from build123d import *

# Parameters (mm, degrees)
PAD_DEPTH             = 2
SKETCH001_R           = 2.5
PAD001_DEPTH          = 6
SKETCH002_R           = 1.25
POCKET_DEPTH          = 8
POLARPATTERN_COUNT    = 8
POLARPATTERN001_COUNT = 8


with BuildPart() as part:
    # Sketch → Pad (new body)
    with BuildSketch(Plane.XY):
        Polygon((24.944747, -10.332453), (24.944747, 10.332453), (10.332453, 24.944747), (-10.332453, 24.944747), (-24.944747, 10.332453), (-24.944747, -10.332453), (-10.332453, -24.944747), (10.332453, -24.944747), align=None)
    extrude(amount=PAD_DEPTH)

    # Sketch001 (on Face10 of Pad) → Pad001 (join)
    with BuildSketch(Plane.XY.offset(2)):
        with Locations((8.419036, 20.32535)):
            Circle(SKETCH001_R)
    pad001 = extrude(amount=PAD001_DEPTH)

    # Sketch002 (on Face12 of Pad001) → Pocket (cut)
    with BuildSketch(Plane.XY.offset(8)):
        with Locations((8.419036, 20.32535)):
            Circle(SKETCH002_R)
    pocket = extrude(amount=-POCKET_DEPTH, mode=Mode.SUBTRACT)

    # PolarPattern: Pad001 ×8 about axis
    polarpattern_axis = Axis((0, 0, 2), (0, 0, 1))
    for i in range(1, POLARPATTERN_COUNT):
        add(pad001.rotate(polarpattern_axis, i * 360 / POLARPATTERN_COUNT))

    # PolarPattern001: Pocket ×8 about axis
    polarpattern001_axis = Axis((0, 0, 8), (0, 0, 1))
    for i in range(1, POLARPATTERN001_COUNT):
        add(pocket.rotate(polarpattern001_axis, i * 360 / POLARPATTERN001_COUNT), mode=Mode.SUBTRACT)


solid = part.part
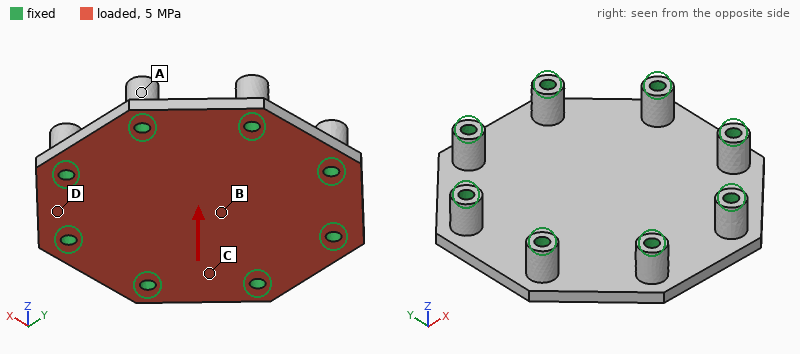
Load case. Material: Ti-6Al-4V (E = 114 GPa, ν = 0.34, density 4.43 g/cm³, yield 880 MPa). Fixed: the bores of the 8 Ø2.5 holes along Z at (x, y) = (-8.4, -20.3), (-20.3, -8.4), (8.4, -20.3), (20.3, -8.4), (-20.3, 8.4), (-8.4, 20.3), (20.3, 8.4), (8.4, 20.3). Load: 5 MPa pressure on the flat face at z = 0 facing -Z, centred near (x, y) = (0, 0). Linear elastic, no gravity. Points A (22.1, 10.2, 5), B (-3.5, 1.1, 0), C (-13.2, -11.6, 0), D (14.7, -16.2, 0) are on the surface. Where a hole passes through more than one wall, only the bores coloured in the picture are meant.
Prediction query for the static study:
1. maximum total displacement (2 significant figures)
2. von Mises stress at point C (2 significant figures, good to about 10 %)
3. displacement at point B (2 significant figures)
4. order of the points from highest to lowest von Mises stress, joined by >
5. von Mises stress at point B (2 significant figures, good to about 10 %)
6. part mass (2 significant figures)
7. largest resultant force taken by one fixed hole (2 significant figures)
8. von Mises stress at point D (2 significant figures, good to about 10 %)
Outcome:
0.21 mm
210 MPa
0.20 mm
B > C > D > A
280 MPa
21 g
1.3 kN
110 MPa
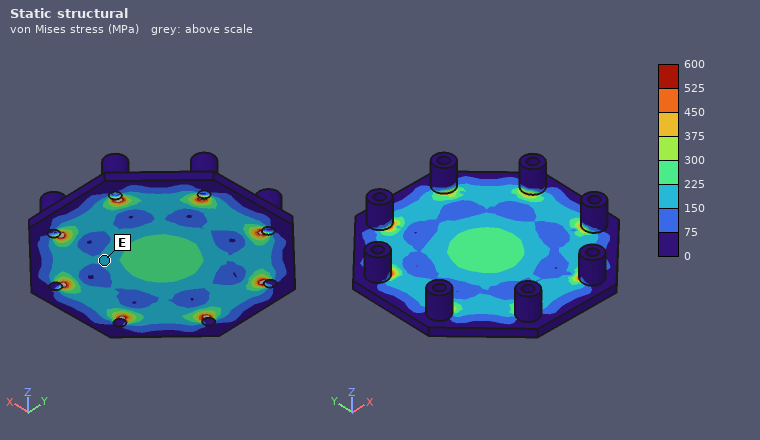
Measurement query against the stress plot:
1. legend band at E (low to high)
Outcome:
150 to 225 MPa
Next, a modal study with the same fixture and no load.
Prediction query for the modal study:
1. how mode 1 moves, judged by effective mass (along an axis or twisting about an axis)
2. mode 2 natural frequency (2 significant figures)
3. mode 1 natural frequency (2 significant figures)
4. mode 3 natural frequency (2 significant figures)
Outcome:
along Z
21 kHz
10 kHz
21 kHz
